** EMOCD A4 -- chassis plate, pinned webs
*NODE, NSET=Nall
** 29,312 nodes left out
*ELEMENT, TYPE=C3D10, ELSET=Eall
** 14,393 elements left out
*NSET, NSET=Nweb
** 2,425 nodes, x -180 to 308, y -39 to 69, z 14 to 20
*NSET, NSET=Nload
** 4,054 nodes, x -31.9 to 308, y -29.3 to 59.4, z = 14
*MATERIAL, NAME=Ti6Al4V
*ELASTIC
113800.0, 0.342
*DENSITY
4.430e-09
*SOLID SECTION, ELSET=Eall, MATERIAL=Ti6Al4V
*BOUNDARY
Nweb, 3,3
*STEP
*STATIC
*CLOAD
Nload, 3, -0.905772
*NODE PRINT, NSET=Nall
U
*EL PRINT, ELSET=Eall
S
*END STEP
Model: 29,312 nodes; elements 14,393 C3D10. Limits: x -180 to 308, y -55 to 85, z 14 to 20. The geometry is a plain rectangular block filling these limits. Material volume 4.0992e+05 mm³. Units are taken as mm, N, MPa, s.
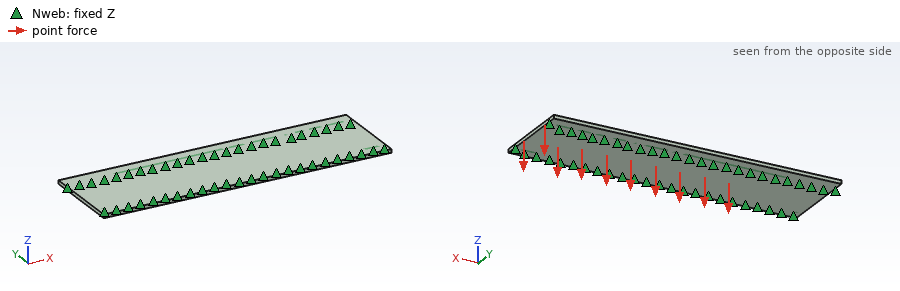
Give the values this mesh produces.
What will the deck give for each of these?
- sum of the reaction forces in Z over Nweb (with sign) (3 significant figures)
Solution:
3670 N
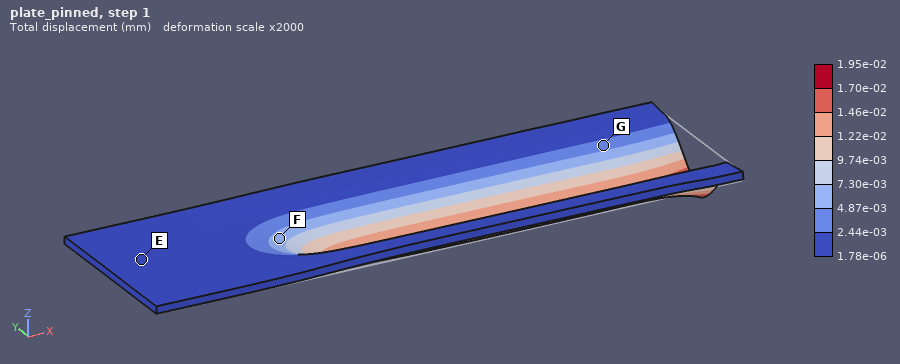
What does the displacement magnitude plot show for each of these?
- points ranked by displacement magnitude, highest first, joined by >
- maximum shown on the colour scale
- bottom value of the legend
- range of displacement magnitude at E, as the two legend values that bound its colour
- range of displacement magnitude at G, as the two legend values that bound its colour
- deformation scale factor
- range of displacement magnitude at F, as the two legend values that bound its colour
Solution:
F > G > E
1.95e-02 mm
1.78e-06 mm
1.78e-06 to 2.44e-03 mm
2.44e-03 to 4.87e-03 mm
2000
4.87e-03 to 7.30e-03 mm
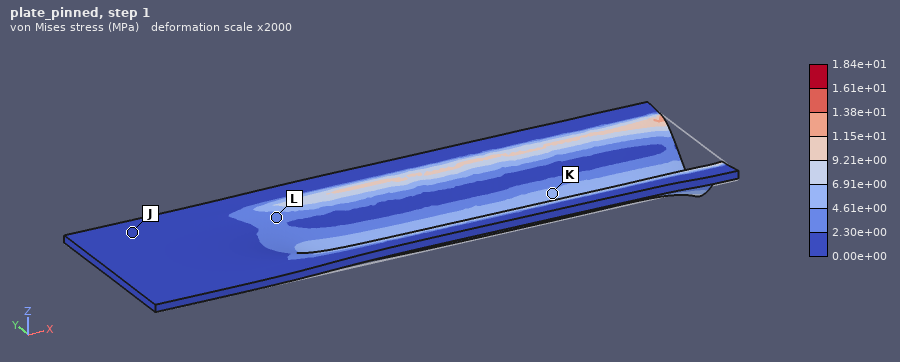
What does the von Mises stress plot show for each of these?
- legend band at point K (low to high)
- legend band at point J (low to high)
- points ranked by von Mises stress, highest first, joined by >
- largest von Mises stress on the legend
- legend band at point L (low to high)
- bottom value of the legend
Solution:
4.61e+00 to 6.91e+00 MPa
0.00e+00 to 2.30e+00 MPa
K > L > J
1.84e+01 MPa
2.30e+00 to 4.61e+00 MPa
0.00e+00 MPa
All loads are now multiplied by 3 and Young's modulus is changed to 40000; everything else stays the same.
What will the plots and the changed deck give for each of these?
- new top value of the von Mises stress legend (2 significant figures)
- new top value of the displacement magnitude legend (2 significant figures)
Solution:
55 MPa
0.17 mm
